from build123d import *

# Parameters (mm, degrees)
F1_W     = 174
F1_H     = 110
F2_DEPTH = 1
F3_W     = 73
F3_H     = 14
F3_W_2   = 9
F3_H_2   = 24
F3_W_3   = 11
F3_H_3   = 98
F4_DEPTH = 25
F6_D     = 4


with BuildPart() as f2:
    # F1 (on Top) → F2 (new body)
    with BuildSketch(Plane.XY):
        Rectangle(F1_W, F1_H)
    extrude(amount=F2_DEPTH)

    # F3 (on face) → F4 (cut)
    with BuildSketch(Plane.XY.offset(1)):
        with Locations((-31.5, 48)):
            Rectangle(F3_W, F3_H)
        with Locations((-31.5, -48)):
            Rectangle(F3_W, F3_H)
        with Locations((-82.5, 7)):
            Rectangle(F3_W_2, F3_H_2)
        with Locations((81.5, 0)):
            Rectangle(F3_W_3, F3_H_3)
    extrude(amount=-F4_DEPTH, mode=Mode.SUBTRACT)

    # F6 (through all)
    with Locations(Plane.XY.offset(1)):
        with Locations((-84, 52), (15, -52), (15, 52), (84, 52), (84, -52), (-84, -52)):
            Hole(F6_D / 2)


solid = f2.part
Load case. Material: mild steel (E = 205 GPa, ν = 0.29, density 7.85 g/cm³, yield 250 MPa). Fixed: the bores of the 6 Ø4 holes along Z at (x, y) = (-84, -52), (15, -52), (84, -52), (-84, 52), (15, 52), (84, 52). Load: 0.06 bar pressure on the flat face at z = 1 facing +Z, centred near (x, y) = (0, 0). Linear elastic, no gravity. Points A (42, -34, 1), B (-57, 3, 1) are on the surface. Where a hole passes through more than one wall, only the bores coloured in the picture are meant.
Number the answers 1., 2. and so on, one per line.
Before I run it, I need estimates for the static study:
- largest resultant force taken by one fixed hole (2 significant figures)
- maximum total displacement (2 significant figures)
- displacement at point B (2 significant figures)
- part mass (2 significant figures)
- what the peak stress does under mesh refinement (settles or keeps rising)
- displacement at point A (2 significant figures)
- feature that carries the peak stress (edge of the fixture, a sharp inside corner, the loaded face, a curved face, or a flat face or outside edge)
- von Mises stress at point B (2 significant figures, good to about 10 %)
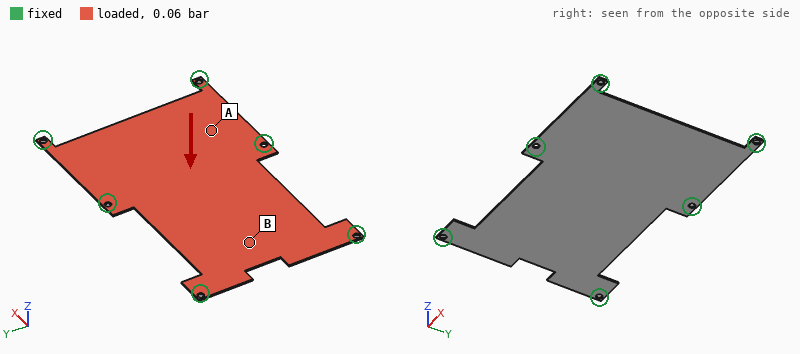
1. 26 N
2. 0.29 mm
3. 0.26 mm
4. 120 g
5. keeps rising
6. 0.11 mm
7. edge of the fixture
8. 21 MPa
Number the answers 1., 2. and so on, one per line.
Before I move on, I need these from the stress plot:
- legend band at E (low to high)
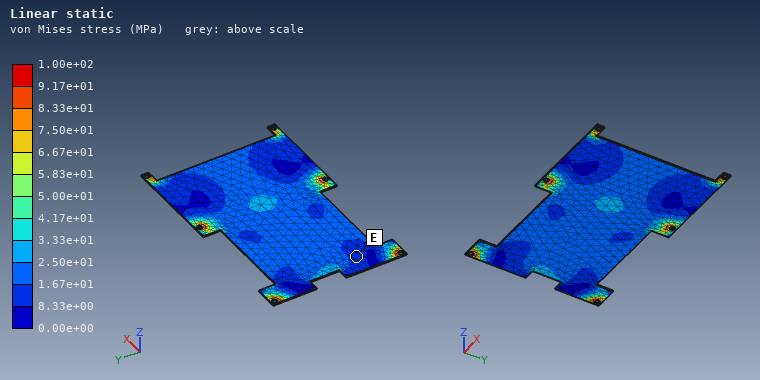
1. 8.33e+00 to 1.67e+01 MPa
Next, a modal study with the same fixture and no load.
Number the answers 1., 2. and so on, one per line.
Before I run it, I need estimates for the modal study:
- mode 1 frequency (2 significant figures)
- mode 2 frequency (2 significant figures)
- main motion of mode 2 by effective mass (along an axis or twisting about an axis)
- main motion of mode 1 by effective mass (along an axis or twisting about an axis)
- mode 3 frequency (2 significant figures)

1. 300 Hz
2. 370 Hz
3. along Z
4. along Z
5. 600 Hz
